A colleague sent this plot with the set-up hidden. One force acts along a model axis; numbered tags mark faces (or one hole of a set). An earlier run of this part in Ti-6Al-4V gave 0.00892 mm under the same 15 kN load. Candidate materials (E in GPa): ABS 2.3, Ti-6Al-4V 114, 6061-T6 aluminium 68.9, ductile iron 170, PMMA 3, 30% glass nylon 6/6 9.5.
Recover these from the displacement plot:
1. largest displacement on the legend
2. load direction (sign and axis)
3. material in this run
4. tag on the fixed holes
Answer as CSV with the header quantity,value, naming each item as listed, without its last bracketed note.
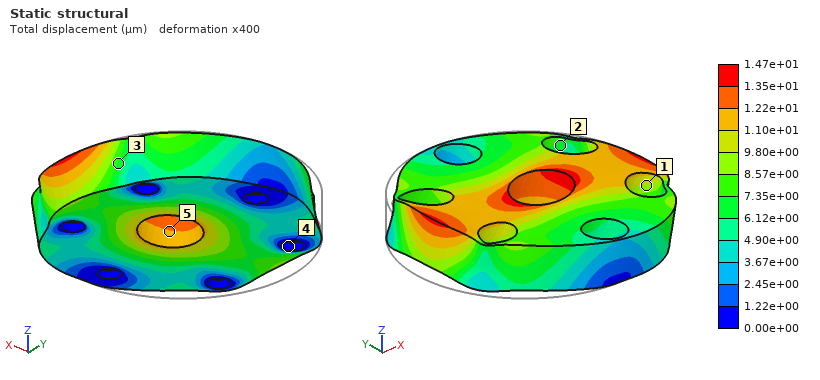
quantity,value
largest displacement on the legend,1.47e+01 µm
load direction,+X
material in this run,6061-T6 aluminium
tag on the fixed holes,4
